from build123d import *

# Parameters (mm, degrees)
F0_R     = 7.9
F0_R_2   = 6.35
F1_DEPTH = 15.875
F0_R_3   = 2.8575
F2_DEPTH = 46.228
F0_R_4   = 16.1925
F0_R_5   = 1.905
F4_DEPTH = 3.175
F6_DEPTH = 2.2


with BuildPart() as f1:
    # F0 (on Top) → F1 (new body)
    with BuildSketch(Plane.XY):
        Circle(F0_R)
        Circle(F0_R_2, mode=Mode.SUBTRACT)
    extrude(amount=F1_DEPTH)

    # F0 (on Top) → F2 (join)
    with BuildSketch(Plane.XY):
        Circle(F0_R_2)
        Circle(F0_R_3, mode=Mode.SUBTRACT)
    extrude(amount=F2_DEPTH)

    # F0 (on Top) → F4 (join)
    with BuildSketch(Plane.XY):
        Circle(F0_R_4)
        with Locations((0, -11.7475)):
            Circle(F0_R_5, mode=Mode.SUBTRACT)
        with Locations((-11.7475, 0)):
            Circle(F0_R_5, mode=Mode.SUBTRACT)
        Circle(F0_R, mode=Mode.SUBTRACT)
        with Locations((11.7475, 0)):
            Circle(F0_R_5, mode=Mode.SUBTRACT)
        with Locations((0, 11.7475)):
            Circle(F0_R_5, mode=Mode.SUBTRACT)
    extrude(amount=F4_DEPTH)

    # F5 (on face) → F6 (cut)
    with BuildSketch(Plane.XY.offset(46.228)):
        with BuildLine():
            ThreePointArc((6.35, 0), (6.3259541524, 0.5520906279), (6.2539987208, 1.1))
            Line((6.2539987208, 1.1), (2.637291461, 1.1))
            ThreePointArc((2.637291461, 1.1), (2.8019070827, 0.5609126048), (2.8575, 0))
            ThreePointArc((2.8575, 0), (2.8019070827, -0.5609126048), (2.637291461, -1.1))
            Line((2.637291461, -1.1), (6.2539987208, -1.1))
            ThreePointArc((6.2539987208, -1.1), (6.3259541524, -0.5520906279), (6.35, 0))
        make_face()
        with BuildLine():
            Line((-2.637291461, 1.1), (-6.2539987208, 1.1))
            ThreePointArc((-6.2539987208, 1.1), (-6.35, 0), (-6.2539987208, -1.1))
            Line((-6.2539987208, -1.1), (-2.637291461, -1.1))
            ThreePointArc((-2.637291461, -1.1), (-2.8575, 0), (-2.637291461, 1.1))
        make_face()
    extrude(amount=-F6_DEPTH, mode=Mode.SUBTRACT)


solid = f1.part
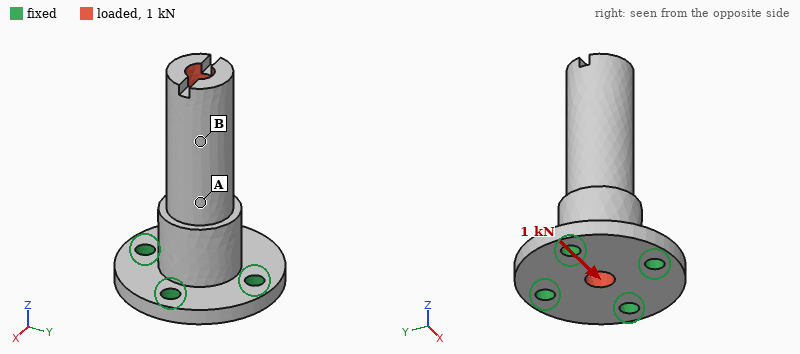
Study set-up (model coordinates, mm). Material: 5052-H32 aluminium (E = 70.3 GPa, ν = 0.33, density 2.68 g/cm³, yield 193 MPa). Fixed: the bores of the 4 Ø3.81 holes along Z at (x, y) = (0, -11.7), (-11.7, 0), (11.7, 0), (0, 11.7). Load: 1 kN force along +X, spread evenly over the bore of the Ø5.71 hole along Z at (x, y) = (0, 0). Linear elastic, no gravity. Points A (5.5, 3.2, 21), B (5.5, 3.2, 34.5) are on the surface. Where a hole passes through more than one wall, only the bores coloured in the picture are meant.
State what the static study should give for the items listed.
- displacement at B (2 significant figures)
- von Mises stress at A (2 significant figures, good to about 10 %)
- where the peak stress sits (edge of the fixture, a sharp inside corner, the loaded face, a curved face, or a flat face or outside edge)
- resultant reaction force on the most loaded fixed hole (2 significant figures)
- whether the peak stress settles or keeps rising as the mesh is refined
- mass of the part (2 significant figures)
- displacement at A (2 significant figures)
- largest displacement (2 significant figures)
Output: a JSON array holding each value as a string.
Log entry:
["0.080 mm", "30 MPa", "edge of the fixture", "1.1 kN", "keeps rising", "20 g", "0.040 mm", "0.12 mm"]
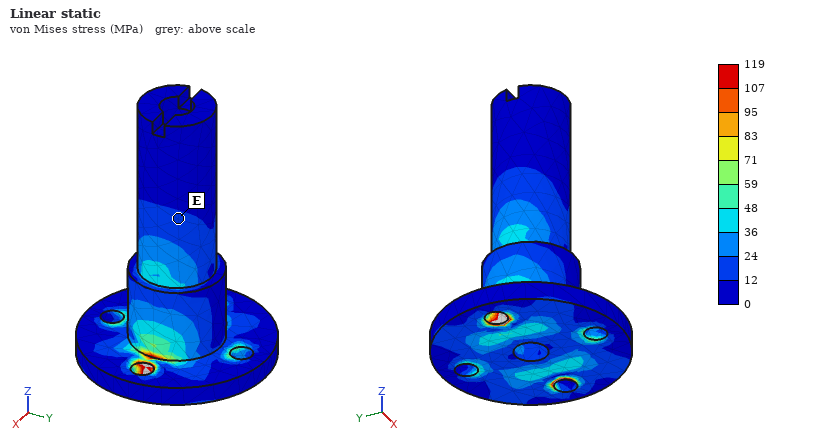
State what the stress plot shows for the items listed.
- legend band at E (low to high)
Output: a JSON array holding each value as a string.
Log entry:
["12 to 24 MPa"]
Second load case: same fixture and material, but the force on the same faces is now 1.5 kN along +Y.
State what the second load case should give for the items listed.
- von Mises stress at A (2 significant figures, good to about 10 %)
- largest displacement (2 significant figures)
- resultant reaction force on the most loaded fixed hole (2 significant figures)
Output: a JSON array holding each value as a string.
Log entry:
["31 MPa", "0.18 mm", "1.7 kN"]
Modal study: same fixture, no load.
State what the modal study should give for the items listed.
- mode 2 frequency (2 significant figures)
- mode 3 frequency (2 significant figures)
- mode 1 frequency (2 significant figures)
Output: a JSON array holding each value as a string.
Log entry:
["5100 Hz", "21 kHz", "5100 Hz"]
